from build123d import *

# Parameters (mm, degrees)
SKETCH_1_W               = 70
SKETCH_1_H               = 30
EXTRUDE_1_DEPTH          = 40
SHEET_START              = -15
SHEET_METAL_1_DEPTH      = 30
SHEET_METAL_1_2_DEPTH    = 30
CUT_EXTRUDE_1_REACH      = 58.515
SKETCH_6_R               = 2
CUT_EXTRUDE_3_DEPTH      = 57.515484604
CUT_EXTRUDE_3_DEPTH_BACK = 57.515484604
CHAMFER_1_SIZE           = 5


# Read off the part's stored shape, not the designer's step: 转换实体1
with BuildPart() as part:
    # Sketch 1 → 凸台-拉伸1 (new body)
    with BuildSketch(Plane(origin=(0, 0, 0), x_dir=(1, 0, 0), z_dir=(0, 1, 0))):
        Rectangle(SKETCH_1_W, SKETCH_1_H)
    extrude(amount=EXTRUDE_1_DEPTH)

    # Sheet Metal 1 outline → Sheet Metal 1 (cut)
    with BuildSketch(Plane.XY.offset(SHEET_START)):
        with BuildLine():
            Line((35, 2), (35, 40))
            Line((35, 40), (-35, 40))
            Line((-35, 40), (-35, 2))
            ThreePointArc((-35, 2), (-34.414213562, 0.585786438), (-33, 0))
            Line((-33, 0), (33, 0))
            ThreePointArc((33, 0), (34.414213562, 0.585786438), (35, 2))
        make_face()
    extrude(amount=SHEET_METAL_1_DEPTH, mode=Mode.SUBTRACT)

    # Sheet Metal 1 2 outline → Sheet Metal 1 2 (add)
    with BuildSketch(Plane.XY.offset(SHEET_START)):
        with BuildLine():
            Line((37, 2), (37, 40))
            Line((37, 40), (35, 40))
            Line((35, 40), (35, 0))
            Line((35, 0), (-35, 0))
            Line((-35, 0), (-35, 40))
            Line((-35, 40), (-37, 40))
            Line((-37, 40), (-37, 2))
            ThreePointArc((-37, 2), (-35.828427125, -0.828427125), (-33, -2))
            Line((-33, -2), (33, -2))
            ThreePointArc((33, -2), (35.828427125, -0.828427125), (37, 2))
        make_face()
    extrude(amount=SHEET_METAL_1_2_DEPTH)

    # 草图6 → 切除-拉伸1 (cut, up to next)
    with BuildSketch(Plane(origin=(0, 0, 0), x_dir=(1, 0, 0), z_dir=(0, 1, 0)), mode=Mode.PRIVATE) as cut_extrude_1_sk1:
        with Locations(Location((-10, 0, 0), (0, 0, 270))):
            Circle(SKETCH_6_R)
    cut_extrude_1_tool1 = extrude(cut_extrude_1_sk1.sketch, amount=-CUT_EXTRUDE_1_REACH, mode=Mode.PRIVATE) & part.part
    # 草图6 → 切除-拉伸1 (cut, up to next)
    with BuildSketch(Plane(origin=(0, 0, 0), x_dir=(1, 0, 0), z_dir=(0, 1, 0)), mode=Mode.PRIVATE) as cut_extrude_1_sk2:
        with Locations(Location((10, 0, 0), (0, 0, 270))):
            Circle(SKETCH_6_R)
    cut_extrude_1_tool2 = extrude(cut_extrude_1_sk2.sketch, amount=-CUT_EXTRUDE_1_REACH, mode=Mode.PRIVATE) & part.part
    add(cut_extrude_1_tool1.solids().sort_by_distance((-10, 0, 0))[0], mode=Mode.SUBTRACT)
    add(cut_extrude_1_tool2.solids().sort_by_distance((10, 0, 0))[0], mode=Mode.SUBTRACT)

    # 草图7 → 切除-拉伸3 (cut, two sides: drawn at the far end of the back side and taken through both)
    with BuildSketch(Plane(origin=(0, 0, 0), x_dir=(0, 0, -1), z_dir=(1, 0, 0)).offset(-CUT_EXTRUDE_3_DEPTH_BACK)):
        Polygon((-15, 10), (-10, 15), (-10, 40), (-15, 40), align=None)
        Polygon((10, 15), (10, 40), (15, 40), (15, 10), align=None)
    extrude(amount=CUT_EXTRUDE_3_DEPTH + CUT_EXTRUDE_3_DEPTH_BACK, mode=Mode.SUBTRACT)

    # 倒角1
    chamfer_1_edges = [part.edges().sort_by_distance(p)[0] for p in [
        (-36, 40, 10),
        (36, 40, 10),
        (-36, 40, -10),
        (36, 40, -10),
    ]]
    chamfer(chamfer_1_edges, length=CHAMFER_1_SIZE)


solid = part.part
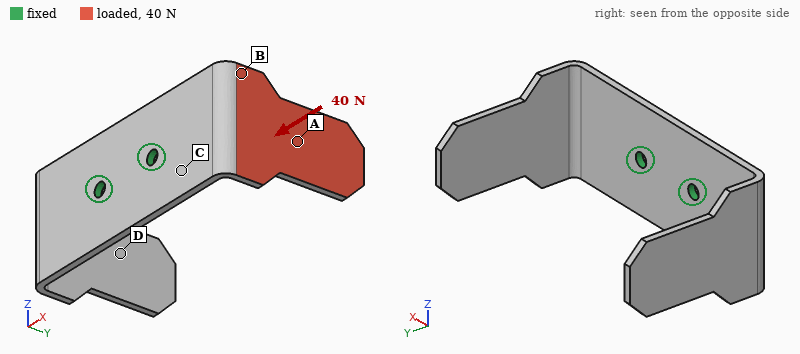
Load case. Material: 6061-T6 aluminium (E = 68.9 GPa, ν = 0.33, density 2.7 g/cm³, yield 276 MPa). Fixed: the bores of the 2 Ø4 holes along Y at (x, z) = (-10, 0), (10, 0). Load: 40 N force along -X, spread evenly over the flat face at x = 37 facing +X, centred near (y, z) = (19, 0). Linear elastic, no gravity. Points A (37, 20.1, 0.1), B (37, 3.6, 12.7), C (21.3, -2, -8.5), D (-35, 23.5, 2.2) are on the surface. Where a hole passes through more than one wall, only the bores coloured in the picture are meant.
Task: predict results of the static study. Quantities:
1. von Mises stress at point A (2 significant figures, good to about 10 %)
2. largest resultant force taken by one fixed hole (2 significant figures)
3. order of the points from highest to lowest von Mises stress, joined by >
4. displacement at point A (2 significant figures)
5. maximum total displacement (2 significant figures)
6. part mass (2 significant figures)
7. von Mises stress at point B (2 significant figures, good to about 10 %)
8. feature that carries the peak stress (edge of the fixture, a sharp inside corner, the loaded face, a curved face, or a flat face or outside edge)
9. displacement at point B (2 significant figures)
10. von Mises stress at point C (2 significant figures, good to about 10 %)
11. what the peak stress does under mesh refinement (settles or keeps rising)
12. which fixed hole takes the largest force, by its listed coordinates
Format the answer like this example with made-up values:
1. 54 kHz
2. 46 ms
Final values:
1. 12 MPa
2. 33 N
3. C > B > A > D
4. 0.43 mm
5. 0.83 mm
6. 21 g
7. 27 MPa
8. edge of the fixture
9. 0.21 mm
10. 36 MPa
11. keeps rising
12. (10, 0)
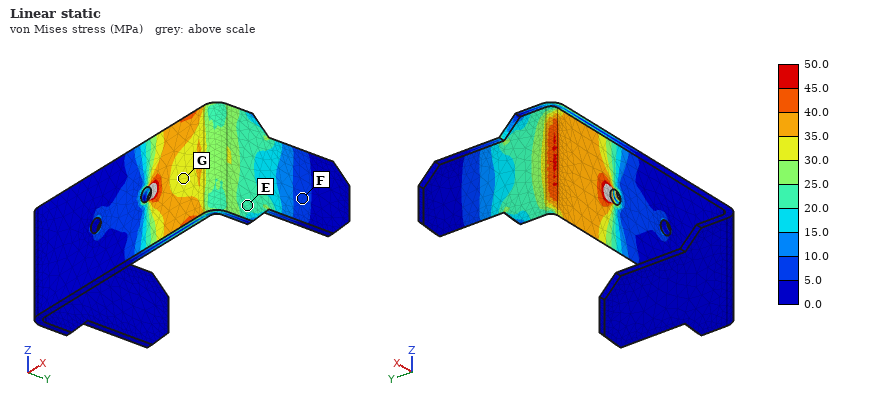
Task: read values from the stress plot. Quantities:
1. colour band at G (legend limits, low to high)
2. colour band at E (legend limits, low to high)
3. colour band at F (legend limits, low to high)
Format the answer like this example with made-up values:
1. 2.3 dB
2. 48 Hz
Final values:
1. 30.0 to 35.0 MPa
2. 20.0 to 25.0 MPa
3. 5.0 to 10.0 MPa
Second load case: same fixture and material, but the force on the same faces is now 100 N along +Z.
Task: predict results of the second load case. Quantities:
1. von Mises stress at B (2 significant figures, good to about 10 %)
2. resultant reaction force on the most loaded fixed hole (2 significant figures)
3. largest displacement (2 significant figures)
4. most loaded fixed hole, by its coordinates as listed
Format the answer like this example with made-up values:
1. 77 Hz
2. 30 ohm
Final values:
1. 37 MPa
2. 210 N
3. 0.91 mm
4. (10, 0)
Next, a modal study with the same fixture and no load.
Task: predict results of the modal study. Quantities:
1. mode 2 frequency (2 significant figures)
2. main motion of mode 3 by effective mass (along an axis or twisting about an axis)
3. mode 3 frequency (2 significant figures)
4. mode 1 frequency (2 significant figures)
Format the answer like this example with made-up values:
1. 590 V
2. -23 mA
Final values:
1. 600 Hz
2. twisting about Y
3. 920 Hz
4. 590 Hz
